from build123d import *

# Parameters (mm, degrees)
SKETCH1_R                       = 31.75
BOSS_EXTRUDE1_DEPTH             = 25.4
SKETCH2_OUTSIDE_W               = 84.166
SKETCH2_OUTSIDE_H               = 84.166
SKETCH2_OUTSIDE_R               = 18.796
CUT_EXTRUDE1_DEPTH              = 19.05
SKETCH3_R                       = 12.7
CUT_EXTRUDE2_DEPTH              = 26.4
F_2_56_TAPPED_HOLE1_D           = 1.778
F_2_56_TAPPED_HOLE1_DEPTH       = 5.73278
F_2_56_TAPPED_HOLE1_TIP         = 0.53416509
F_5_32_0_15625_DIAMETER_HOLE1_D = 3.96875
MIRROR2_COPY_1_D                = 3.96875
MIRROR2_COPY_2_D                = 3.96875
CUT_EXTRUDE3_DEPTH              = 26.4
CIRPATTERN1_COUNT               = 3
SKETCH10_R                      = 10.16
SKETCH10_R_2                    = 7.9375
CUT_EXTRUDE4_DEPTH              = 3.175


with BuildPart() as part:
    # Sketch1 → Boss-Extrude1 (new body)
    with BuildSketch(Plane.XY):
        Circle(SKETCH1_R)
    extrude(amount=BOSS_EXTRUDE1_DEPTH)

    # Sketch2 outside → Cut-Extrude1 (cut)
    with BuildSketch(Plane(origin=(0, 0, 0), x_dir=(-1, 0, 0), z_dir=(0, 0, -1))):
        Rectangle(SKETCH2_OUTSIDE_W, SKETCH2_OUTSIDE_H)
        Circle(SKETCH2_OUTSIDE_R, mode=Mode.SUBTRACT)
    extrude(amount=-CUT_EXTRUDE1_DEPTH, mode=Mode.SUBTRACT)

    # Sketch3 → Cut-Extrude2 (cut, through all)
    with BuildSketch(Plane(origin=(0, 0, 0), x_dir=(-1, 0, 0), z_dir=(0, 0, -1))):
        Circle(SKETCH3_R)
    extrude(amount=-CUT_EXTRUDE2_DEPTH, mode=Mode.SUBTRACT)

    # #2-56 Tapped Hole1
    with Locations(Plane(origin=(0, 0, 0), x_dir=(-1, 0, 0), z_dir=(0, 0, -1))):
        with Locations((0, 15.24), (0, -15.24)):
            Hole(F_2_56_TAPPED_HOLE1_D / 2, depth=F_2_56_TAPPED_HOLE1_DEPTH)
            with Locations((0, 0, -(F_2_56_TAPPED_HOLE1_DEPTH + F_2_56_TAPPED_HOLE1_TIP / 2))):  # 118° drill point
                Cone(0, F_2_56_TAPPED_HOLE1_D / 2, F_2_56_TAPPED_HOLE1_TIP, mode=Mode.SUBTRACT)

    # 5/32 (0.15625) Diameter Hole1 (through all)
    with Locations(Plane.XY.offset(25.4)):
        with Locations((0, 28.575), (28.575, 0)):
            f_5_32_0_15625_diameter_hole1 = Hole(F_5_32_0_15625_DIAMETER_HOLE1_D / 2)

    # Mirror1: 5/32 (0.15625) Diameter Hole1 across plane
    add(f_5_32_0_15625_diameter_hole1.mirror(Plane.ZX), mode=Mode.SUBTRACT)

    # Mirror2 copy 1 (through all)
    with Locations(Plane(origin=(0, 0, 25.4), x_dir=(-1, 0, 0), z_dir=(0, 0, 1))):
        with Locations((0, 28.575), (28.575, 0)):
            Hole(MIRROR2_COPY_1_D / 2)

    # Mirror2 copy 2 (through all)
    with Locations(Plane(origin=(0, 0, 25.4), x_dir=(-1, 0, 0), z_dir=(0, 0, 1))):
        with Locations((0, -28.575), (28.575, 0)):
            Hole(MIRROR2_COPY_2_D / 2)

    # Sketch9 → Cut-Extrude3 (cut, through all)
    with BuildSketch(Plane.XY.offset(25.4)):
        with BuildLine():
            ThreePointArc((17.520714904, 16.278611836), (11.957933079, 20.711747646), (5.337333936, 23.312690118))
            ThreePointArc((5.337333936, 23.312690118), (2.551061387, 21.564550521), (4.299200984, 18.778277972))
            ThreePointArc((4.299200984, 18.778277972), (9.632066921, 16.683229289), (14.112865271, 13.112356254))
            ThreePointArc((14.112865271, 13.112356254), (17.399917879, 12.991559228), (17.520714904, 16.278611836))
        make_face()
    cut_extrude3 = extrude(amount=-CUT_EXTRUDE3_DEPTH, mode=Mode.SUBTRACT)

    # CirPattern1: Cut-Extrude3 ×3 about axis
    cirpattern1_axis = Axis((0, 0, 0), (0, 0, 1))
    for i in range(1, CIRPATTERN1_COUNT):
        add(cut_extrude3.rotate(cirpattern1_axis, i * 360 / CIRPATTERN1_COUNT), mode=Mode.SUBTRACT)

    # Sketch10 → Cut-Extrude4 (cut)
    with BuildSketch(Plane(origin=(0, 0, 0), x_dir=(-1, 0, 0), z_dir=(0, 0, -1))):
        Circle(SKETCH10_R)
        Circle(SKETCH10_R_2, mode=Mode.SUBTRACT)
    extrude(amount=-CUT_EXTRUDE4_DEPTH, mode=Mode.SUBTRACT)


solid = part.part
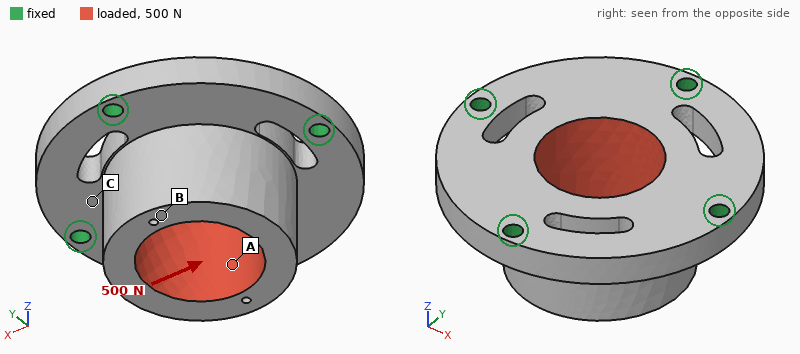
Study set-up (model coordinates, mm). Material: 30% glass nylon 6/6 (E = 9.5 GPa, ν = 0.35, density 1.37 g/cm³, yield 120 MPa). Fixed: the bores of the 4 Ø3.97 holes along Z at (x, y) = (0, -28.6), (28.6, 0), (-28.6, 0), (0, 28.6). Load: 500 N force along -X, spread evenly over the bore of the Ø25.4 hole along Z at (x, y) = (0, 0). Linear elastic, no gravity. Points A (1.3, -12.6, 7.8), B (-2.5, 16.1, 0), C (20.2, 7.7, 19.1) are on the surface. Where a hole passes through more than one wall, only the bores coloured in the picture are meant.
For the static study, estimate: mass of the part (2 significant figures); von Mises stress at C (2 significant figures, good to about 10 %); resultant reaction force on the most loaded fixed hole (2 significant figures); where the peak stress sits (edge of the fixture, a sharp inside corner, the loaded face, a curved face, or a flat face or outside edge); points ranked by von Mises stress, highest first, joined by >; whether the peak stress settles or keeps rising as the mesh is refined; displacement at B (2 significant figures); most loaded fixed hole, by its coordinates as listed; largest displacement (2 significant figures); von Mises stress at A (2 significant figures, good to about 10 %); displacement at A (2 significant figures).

36 g
3.2 MPa
220 N
edge of the fixture
C > A > B
keeps rising
19 µm
(28.6, 0)
27 µm
1.5 MPa
14 µm
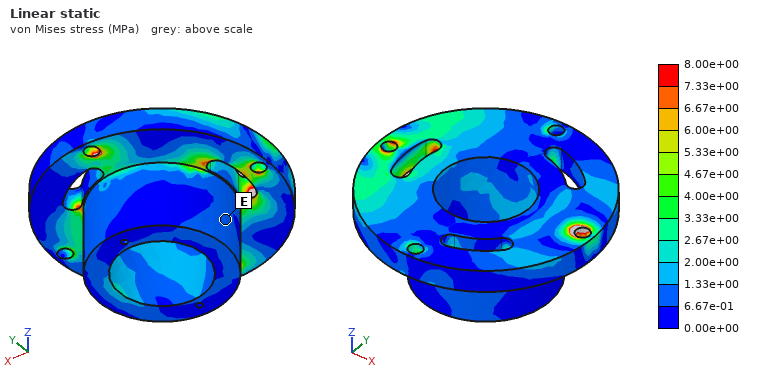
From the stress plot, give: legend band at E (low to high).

6.67e-01 to 1.33e+00 MPa
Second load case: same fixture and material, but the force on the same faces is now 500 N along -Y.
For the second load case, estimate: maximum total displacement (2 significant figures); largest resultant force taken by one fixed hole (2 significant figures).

19 µm
170 N
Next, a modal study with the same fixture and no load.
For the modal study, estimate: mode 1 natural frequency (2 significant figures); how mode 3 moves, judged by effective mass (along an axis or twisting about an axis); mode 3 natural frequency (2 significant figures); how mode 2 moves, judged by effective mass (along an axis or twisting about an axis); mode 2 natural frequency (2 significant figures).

4700 Hz
along Z
6200 Hz
along Y
5900 Hz
